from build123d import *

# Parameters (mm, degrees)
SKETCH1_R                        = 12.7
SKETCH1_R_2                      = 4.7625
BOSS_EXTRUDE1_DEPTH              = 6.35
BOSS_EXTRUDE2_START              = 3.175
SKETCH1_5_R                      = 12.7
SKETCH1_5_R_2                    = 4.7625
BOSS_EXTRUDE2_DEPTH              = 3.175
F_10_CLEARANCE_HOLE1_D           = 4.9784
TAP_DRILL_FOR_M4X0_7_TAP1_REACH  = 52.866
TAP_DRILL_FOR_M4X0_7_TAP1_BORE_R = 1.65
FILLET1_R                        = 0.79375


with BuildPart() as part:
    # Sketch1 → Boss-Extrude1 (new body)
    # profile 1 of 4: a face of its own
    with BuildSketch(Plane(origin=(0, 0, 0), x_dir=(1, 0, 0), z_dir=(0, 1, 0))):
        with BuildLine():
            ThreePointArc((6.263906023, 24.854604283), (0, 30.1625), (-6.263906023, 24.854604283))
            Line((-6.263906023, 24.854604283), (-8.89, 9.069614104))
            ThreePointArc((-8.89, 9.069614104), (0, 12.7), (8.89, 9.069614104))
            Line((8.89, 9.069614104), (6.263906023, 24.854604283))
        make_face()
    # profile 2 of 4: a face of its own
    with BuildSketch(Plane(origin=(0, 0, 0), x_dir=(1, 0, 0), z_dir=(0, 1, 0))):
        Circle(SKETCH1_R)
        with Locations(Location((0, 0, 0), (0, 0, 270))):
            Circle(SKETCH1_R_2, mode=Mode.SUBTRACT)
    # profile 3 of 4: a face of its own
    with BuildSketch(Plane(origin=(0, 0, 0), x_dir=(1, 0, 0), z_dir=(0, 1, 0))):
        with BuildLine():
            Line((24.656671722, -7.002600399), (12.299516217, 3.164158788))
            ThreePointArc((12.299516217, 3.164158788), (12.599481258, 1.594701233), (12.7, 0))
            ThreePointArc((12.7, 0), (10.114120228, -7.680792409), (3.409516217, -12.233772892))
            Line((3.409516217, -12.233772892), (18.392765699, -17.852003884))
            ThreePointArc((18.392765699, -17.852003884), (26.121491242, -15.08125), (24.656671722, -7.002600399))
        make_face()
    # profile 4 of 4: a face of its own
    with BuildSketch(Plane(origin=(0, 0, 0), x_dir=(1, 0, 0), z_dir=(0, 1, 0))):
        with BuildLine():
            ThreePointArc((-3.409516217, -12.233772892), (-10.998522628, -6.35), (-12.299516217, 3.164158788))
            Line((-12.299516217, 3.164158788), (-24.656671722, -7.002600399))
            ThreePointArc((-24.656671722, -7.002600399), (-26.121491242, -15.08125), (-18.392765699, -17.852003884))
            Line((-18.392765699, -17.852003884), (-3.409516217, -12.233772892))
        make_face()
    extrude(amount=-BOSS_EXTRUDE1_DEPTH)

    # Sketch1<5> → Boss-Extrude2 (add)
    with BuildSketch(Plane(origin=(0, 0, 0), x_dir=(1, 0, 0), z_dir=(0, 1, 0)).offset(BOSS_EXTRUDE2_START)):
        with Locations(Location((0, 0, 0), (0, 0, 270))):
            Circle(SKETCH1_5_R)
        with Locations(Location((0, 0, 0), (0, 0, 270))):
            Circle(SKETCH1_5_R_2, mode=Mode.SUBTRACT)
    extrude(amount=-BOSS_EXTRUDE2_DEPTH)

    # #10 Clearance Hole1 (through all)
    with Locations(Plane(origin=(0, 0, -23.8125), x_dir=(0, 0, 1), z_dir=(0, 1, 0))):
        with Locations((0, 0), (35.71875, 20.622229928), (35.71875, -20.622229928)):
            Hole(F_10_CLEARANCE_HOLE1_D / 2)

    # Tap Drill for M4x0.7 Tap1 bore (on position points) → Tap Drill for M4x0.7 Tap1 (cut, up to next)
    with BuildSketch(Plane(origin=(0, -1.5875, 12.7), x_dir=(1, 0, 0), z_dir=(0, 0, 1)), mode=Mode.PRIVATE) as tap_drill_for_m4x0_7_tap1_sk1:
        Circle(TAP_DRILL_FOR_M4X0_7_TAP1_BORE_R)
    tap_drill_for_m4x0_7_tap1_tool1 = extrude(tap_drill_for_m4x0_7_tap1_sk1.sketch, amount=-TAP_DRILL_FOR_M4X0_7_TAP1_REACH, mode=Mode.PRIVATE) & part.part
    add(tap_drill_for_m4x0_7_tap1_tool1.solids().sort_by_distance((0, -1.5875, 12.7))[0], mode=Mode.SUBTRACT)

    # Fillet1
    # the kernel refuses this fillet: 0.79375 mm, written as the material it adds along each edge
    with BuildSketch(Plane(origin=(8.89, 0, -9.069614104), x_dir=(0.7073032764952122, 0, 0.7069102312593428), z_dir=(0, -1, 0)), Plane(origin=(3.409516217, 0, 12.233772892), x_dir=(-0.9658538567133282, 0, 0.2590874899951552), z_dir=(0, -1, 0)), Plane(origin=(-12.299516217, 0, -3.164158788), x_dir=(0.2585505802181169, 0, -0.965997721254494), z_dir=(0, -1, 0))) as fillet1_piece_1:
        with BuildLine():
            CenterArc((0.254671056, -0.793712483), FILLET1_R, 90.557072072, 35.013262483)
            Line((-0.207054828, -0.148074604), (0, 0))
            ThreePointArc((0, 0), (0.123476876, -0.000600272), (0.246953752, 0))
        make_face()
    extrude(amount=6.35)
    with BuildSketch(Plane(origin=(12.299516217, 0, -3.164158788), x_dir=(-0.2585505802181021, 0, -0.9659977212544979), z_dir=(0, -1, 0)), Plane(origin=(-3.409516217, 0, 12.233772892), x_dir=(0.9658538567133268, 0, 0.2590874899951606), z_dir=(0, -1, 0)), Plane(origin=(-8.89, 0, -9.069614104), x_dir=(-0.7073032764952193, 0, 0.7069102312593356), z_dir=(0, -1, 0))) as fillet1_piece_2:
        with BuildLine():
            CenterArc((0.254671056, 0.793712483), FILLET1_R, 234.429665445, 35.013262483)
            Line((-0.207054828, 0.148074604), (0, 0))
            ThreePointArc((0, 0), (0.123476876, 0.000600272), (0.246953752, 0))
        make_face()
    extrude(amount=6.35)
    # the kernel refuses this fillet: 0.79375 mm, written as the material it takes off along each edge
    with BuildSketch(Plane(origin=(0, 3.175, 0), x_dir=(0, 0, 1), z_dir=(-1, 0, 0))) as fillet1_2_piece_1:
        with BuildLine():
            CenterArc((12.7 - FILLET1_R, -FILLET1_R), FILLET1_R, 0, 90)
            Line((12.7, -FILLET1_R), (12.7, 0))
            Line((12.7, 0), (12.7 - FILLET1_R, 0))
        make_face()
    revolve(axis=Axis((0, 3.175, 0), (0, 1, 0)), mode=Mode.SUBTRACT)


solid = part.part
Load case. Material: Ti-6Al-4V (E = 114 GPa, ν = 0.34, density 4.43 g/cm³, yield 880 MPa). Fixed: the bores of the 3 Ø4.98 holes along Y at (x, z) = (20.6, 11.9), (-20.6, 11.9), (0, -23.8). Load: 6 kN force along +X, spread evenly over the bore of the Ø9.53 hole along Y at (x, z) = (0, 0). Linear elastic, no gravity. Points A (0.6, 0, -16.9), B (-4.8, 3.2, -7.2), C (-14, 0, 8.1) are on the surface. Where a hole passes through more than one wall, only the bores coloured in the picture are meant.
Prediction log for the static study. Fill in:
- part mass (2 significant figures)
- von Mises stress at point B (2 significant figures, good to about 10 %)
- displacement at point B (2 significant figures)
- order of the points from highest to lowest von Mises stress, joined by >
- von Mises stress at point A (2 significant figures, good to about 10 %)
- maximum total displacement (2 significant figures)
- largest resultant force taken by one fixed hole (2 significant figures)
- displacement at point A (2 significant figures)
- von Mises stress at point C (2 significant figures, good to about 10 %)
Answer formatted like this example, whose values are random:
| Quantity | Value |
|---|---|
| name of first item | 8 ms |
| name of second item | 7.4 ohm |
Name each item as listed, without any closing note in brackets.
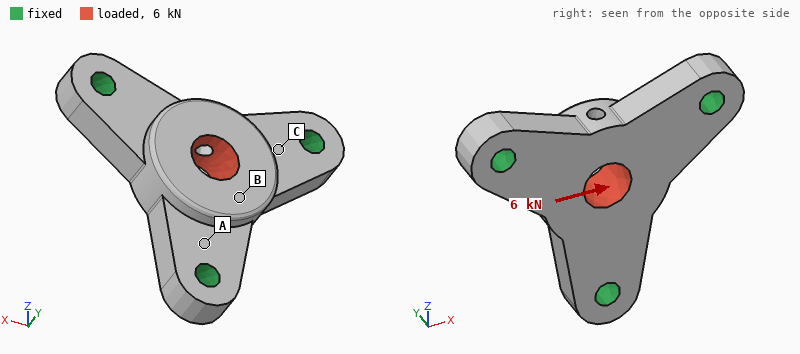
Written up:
| Quantity | Value |
|---|---|
| part mass | 37 g |
| von Mises stress at point B | 12 MPa |
| displacement at point B | 9.5 µm |
| order of the points from highest to lowest von Mises stress, joined by > | C > A > B |
| von Mises stress at point A | 24 MPa |
| maximum total displacement | 11 µm |
| largest resultant force taken by one fixed hole | 2.9 kN |
| displacement at point A | 3.3 µm |
| von Mises stress at point C | 44 MPa |
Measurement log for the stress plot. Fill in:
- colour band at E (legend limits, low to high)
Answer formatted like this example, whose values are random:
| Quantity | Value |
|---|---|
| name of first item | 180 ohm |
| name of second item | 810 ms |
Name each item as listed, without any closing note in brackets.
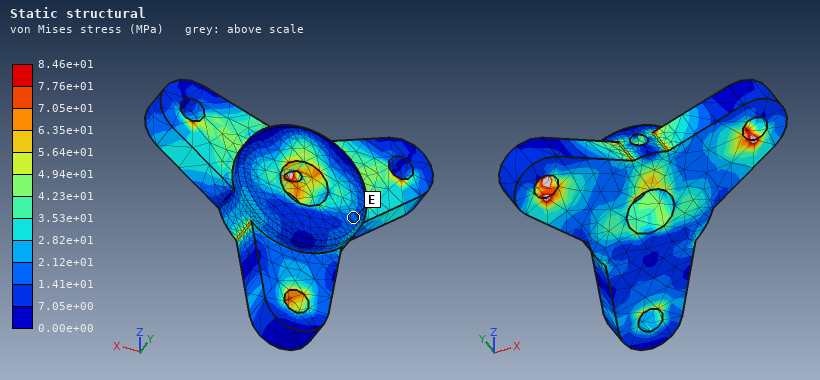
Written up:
| Quantity | Value |
|---|---|
| colour band at E | 1.41e+01 to 2.12e+01 MPa |
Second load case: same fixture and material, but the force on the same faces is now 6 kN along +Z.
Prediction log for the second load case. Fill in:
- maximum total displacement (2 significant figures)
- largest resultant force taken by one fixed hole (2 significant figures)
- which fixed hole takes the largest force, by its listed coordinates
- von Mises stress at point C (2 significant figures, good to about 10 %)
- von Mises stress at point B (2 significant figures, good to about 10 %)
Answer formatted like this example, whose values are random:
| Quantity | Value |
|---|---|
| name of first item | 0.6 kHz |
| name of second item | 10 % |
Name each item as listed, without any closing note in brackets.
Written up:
| Quantity | Value |
|---|---|
| maximum total displacement | 11 µm |
| largest resultant force taken by one fixed hole | 3.3 kN |
| which fixed hole takes the largest force, by its listed coordinates | (0, -23.8) |
| von Mises stress at point C | 31 MPa |
| von Mises stress at point B | 29 MPa |
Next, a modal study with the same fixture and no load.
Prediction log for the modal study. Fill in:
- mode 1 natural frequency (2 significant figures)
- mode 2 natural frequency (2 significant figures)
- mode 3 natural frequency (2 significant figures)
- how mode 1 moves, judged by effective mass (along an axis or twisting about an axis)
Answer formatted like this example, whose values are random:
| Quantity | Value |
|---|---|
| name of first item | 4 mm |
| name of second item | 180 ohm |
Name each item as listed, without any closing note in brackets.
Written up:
| Quantity | Value |
|---|---|
| mode 1 natural frequency | 17 kHz |
| mode 2 natural frequency | 27 kHz |
| mode 3 natural frequency | 27 kHz |
| how mode 1 moves, judged by effective mass | along Y |
